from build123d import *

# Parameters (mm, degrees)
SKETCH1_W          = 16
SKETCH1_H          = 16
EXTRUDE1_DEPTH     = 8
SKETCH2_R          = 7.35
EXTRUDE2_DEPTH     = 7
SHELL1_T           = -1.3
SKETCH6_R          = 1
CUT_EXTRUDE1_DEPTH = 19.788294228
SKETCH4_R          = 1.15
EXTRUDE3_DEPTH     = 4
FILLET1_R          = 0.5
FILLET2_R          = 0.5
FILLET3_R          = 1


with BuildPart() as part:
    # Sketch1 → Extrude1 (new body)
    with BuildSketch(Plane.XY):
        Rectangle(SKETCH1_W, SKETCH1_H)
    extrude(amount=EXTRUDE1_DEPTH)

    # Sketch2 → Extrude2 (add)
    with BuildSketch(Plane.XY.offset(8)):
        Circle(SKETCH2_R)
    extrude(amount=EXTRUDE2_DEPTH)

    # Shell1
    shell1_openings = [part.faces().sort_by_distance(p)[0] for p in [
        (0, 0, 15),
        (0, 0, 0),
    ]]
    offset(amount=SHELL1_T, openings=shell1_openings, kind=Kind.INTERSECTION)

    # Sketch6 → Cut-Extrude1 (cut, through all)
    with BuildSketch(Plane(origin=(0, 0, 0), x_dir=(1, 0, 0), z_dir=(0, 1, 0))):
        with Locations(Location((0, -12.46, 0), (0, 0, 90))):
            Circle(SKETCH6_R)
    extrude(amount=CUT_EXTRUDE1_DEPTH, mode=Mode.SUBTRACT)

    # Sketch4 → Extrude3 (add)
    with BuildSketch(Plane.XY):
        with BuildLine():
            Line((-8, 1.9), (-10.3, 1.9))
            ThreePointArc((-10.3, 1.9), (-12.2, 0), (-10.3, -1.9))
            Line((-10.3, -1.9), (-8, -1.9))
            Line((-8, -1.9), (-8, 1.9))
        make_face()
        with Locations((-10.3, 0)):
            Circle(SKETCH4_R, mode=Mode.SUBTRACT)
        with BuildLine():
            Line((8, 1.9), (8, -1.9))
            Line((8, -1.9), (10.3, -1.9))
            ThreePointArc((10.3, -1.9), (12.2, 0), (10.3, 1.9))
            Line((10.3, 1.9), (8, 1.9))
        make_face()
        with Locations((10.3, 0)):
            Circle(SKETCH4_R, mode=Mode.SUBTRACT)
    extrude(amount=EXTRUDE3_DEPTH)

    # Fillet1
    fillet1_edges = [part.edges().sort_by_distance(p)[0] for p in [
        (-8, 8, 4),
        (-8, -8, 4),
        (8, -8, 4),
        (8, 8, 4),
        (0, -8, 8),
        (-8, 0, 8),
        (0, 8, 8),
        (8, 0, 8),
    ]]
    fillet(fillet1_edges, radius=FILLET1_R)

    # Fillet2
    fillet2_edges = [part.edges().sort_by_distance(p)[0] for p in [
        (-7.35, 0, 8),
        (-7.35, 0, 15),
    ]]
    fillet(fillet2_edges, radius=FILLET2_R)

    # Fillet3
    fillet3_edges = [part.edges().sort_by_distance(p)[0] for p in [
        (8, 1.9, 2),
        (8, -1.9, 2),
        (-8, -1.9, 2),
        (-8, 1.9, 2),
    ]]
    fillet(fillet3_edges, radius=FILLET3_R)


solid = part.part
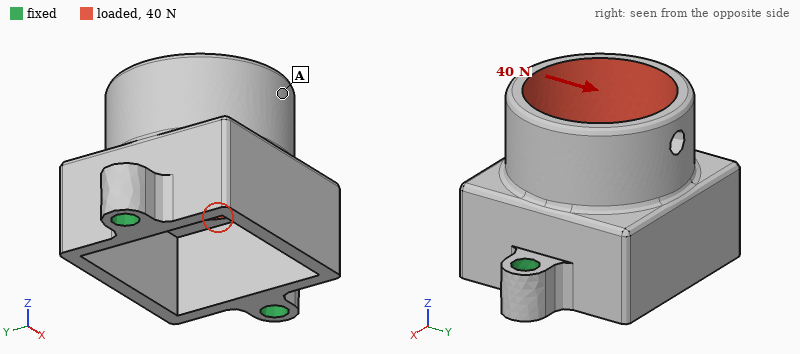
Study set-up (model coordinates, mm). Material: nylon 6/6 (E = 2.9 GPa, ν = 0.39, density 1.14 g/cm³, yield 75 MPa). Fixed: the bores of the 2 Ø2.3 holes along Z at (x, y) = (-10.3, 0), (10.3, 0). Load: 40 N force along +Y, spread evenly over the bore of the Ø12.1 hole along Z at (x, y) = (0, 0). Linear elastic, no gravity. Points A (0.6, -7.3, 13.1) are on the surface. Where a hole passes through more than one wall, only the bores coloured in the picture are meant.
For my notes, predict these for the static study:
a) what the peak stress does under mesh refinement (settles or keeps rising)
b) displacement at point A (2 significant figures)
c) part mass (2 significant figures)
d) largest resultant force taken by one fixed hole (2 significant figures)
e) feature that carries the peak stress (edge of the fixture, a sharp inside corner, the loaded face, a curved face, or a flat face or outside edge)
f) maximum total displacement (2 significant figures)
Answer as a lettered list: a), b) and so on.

a) keeps rising
b) 0.16 mm
c) 1.3 g
d) 20 N
e) edge of the fixture
f) 0.17 mm
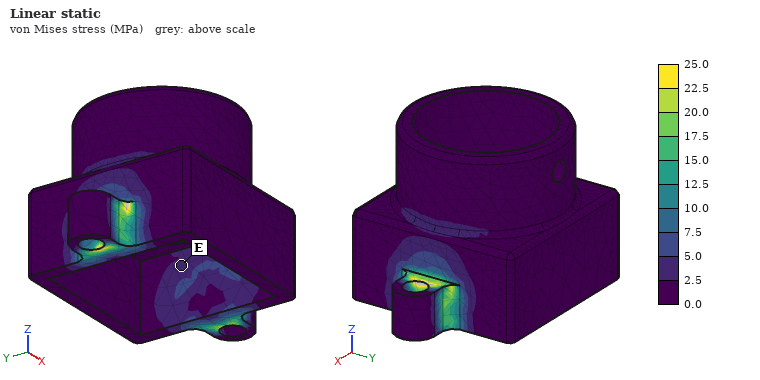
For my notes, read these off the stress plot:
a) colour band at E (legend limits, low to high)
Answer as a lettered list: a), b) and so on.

a) 2.5 to 5.0 MPa
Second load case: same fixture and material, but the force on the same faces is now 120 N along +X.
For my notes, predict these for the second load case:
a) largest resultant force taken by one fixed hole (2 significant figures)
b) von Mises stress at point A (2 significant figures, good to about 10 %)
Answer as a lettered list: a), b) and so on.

a) 80 N
b) 2.4 MPa
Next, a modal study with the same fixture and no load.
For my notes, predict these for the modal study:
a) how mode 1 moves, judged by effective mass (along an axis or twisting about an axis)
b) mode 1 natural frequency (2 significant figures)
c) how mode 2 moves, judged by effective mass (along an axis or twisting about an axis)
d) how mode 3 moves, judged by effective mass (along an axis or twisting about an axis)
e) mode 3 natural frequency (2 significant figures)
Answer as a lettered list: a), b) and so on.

a) along Y
b) 3000 Hz
c) along X
d) twisting about Z
e) 5700 Hz
